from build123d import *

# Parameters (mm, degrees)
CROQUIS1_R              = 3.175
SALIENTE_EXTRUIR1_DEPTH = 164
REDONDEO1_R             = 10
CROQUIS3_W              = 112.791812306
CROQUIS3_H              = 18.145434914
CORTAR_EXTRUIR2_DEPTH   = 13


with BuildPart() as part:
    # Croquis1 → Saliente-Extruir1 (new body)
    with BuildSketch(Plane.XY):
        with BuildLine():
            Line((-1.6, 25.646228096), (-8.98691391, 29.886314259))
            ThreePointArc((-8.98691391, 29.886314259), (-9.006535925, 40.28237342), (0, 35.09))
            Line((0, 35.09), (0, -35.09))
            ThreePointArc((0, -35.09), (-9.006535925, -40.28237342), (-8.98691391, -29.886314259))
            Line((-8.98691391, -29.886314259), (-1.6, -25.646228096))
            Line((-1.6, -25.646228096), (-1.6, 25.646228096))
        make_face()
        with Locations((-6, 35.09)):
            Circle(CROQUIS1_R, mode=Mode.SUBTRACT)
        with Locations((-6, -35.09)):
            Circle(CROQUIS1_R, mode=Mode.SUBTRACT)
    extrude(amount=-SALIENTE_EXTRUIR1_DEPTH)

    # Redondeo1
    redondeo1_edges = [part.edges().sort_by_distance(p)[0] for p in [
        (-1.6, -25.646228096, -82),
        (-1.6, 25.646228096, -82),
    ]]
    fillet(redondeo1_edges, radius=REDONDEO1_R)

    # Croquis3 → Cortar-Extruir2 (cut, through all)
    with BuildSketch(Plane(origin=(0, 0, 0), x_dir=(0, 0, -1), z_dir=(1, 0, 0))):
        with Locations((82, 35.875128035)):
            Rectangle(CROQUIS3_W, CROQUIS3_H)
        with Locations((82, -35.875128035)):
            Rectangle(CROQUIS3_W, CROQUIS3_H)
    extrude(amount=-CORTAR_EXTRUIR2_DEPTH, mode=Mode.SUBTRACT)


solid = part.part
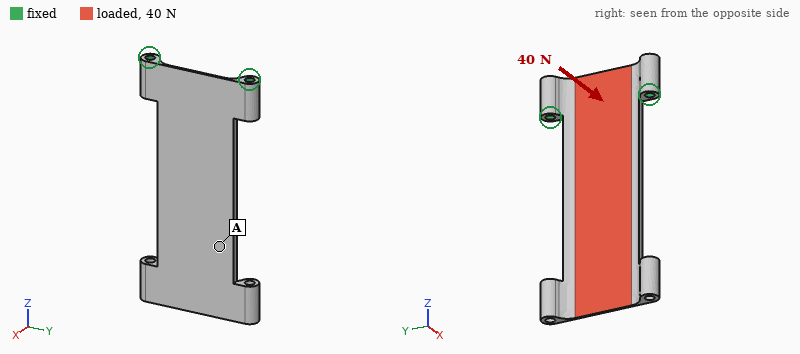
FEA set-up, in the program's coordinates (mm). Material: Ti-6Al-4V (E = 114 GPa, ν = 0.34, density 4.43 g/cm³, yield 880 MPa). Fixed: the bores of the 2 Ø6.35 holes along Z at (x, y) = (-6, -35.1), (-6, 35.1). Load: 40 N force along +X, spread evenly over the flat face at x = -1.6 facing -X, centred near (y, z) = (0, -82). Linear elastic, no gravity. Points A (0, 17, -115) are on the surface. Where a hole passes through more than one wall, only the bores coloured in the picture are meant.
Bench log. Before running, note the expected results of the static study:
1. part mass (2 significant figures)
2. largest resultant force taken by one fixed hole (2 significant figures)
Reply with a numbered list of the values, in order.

1. 120 g
2. 29 N
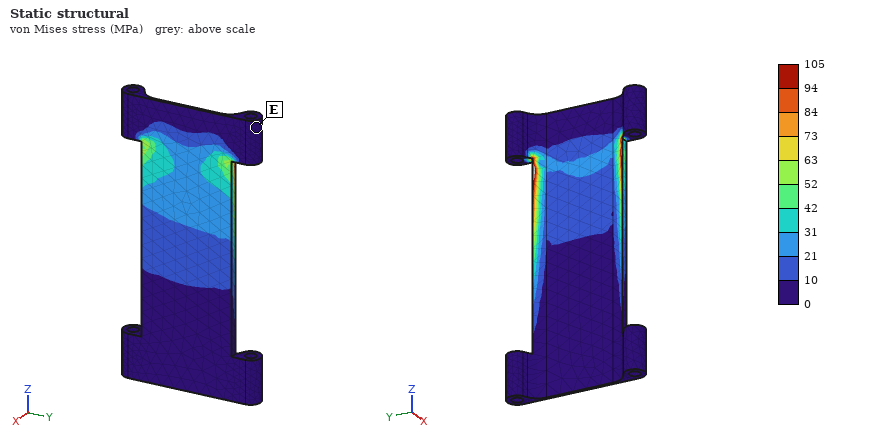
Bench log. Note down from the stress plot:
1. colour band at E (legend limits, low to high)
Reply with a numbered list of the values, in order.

1. 0 to 10 MPa
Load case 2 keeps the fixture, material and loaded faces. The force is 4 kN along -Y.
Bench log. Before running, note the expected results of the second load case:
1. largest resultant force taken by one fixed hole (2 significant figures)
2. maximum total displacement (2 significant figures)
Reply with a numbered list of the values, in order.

1. 5.2 kN
2. 2.2 mm
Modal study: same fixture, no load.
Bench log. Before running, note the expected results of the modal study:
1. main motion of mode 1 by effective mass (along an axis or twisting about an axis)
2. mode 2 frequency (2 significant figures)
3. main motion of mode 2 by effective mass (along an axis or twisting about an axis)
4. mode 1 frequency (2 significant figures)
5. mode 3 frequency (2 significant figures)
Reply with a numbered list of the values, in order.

1. along X
2. 190 Hz
3. twisting about Z
4. 71 Hz
5. 550 Hz
